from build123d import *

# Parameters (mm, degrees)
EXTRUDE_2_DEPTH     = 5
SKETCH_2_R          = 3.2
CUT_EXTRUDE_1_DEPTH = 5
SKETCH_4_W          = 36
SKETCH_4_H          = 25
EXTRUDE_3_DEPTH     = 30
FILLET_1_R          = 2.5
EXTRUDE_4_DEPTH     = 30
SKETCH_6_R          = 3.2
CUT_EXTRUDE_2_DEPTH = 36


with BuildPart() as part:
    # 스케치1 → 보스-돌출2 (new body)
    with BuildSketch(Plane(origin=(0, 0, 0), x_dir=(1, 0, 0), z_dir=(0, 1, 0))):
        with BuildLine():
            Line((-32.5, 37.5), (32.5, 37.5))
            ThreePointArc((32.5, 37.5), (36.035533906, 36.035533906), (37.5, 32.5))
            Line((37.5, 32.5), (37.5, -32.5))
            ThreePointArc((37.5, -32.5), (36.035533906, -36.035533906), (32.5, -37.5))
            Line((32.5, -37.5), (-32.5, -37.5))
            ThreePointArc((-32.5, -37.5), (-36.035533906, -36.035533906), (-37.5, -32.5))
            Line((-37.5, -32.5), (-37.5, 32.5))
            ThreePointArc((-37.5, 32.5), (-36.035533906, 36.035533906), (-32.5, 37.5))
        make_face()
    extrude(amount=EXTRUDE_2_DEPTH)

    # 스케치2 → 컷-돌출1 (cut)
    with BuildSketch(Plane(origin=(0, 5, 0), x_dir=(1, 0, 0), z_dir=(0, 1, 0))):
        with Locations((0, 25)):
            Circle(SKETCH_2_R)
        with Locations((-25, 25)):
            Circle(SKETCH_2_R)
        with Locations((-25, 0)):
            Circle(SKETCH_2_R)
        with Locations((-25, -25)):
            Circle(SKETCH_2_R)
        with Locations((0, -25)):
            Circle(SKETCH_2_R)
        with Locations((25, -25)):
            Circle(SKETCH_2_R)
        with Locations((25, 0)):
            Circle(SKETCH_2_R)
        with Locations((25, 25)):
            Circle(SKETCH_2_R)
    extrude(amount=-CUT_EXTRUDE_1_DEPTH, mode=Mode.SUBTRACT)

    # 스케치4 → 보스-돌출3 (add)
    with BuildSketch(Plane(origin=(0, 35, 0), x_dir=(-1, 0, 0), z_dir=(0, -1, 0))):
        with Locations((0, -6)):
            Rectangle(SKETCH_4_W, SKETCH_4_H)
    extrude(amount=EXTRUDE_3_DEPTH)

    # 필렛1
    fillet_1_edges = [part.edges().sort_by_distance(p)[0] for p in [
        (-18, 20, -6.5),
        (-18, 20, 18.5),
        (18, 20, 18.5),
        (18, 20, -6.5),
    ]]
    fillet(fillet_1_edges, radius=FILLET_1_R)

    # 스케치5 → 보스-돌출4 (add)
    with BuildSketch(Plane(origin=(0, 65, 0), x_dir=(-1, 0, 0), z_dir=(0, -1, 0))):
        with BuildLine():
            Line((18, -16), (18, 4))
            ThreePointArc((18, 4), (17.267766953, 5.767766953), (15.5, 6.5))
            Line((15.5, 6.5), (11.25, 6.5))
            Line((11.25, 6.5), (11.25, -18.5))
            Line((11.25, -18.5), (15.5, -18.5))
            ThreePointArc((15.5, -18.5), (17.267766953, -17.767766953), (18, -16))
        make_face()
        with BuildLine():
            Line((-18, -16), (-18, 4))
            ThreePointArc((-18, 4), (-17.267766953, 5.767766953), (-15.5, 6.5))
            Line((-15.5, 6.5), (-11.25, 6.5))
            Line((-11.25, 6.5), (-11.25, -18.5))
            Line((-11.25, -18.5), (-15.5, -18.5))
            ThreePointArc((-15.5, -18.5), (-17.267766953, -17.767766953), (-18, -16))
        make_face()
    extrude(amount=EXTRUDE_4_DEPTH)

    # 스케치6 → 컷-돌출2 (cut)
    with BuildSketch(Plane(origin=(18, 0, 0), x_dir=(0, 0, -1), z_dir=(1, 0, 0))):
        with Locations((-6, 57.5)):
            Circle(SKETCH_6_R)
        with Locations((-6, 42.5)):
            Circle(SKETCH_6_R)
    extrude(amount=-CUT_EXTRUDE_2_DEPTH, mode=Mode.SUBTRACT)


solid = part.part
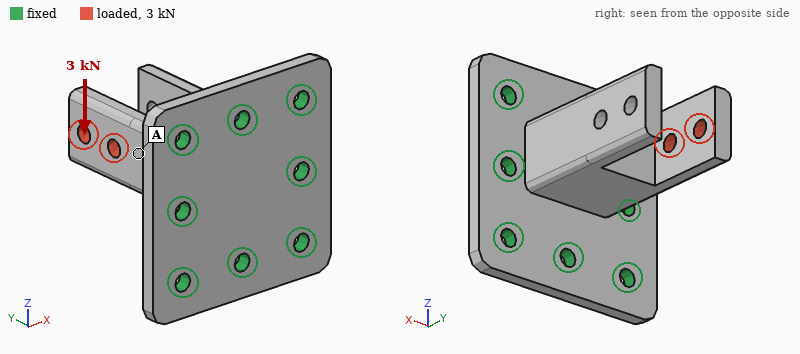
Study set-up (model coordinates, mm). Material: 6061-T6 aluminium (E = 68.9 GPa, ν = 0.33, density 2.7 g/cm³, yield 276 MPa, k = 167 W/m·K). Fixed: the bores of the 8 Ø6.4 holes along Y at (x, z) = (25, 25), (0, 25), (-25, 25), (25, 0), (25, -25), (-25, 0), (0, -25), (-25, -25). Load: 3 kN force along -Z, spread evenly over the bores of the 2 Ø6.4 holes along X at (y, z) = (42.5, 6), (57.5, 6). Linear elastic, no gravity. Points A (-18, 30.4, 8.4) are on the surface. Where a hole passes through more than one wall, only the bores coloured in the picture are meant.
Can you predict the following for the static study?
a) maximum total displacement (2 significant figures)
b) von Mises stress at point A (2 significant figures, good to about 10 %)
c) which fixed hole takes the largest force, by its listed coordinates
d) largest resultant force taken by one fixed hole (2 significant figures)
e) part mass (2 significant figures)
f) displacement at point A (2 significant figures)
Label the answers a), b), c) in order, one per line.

a) 0.23 mm
b) 17 MPa
c) (0, 25)
d) 3.7 kN
e) 170 g
f) 0.068 mm
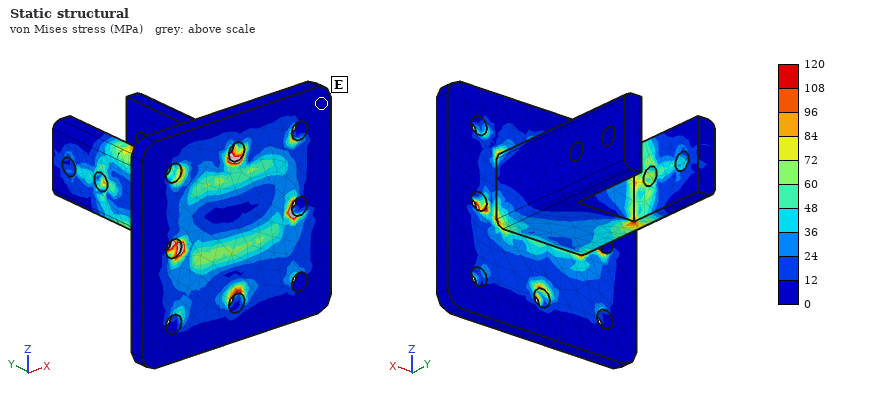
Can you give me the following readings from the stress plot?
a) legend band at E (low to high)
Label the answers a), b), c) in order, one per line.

a) 0 to 12 MPa
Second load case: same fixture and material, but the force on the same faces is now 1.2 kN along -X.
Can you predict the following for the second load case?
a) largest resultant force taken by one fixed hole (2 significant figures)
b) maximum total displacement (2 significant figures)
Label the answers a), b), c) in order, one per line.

a) 1.1 kN
b) 0.20 mm
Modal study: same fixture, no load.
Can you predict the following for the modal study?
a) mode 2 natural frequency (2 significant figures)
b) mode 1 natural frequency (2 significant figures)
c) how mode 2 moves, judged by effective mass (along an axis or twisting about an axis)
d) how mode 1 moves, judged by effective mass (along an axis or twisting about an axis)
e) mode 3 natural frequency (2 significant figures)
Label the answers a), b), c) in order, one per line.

a) 4200 Hz
b) 3900 Hz
c) along Z
d) along X
e) 4600 Hz
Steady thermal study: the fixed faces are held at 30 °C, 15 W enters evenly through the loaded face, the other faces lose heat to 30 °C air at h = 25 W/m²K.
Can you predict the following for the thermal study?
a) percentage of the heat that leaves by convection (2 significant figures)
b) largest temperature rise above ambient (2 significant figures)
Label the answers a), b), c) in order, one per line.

a) 8.1 %
b) 17 K
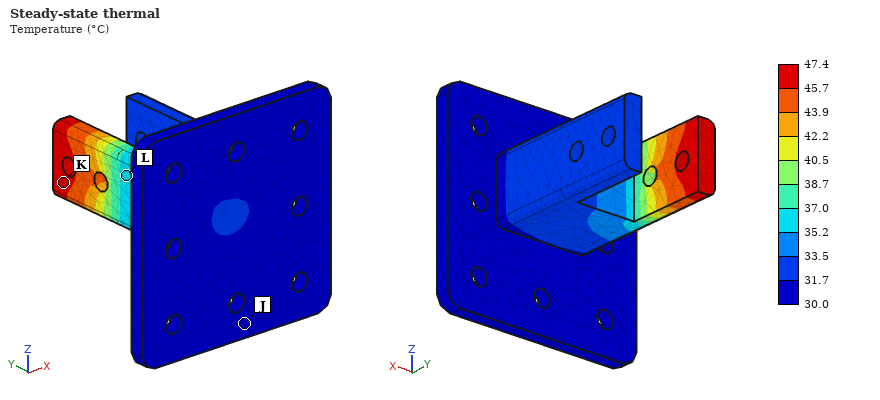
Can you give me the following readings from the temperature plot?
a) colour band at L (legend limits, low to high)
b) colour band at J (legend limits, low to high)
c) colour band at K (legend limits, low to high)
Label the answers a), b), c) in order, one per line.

a) 35.2 to 37.0 °C
b) 30.0 to 31.7 °C
c) 45.7 to 47.4 °C
